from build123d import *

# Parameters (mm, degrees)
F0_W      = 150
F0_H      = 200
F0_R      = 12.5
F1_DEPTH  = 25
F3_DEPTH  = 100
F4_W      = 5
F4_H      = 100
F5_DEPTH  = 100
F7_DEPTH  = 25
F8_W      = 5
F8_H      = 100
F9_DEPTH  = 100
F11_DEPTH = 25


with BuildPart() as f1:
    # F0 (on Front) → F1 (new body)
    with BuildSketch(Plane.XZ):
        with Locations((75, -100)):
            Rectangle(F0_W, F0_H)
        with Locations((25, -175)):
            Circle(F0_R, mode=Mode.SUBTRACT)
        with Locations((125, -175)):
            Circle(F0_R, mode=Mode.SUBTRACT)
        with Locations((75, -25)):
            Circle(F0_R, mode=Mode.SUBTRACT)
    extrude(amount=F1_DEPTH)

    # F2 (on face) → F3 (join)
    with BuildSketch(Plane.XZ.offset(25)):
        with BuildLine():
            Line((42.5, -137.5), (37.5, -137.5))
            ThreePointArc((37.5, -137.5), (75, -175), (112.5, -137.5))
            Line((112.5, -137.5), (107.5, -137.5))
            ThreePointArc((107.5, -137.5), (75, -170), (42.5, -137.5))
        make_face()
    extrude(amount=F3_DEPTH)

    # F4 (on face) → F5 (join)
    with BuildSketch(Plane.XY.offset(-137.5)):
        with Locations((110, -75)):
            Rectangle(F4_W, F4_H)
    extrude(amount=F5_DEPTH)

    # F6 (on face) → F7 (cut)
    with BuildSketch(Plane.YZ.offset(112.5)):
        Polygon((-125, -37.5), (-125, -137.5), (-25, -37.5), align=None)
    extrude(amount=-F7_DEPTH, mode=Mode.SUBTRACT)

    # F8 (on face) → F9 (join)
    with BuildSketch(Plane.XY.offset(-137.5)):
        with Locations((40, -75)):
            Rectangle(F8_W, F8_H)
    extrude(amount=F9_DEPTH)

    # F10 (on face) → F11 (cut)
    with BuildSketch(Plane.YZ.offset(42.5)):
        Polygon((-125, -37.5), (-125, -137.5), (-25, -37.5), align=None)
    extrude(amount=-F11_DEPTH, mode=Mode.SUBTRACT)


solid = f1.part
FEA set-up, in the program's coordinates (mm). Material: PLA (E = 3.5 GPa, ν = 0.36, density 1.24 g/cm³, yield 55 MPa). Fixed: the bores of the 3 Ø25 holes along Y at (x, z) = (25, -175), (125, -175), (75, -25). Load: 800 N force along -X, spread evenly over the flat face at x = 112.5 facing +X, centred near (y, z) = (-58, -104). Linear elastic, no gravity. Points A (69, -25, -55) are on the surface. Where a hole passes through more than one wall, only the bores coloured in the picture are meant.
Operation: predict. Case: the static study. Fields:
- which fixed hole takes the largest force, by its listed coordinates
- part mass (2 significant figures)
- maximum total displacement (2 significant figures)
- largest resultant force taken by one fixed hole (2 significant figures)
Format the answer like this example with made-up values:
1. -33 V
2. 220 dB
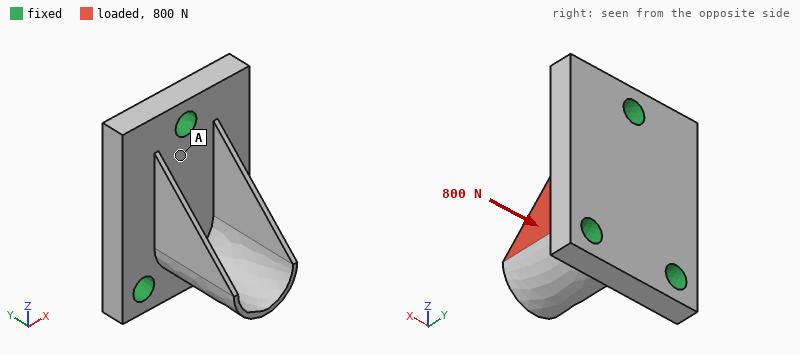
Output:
1. (125, -175)
2. 1.0 kg
3. 2.6 mm
4. 500 N
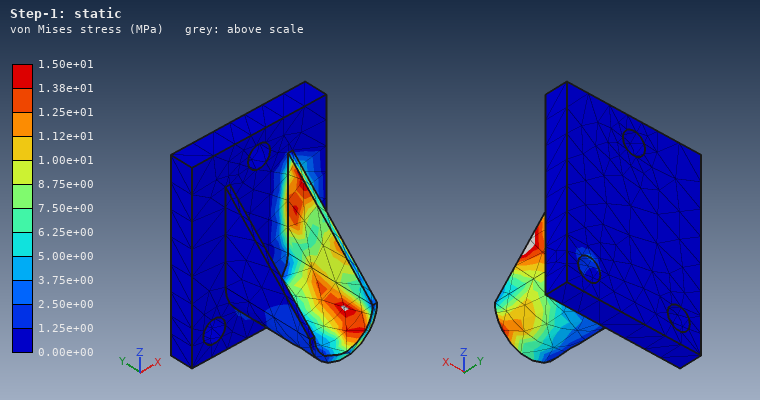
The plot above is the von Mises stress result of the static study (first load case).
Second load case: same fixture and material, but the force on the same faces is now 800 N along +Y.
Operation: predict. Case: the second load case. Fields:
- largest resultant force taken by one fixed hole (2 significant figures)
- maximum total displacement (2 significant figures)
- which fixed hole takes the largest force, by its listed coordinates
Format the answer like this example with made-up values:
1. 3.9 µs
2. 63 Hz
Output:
1. 460 N
2. 0.28 mm
3. (125, -175)
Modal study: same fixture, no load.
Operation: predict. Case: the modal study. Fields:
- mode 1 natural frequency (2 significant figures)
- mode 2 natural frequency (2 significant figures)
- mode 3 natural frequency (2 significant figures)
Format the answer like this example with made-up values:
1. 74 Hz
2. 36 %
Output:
1. 570 Hz
2. 670 Hz
3. 1100 Hz
